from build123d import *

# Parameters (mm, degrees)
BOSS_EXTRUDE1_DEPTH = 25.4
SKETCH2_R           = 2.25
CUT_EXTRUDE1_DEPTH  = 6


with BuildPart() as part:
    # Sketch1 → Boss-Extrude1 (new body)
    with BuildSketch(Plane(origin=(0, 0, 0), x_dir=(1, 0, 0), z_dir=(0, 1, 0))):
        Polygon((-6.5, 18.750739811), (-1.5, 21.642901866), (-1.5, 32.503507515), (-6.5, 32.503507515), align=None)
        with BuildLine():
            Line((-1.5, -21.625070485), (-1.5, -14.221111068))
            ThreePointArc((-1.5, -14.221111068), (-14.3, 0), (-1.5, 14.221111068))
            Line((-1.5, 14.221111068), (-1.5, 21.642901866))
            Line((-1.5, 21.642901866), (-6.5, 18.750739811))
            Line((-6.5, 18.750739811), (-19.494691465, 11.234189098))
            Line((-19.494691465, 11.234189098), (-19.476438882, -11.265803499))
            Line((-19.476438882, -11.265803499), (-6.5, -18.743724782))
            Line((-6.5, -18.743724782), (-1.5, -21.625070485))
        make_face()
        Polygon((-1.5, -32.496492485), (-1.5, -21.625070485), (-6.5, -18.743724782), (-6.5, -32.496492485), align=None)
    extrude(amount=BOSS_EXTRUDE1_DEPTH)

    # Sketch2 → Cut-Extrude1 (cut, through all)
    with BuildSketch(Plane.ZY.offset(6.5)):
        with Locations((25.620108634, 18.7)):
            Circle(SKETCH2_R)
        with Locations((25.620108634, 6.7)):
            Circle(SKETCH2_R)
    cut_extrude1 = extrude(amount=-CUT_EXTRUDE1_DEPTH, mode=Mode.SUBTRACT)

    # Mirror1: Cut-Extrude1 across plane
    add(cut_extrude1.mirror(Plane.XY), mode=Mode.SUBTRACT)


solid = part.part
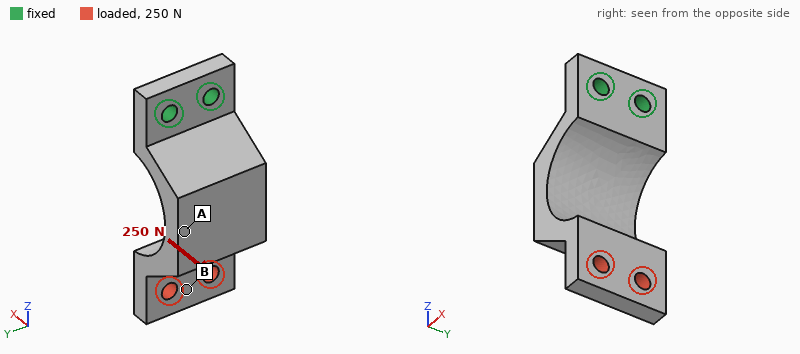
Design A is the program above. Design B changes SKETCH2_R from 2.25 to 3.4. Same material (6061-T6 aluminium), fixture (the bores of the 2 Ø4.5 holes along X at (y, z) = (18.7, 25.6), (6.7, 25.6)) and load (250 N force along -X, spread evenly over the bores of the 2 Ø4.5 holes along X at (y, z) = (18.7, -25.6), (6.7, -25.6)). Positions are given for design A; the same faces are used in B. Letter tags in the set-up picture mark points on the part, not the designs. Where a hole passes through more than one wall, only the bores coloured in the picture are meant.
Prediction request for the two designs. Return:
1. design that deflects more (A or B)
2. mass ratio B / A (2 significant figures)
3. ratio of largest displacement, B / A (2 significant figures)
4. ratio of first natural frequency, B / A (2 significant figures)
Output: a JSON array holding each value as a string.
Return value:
["A", "0.96", "0.92", "1.1"]
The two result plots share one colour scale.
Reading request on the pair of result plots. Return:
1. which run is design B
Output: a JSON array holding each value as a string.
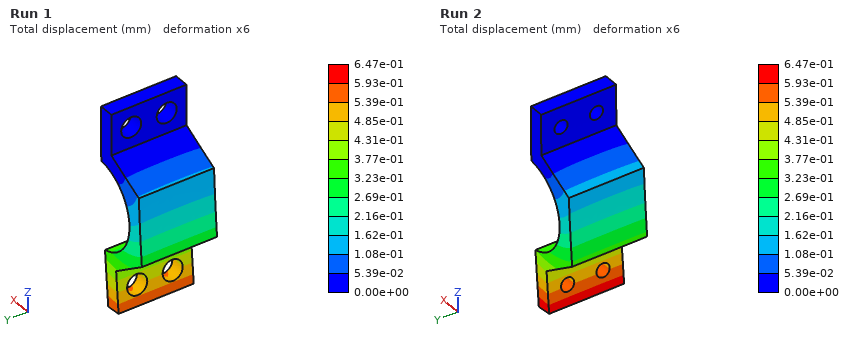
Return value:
["Run 1"]
